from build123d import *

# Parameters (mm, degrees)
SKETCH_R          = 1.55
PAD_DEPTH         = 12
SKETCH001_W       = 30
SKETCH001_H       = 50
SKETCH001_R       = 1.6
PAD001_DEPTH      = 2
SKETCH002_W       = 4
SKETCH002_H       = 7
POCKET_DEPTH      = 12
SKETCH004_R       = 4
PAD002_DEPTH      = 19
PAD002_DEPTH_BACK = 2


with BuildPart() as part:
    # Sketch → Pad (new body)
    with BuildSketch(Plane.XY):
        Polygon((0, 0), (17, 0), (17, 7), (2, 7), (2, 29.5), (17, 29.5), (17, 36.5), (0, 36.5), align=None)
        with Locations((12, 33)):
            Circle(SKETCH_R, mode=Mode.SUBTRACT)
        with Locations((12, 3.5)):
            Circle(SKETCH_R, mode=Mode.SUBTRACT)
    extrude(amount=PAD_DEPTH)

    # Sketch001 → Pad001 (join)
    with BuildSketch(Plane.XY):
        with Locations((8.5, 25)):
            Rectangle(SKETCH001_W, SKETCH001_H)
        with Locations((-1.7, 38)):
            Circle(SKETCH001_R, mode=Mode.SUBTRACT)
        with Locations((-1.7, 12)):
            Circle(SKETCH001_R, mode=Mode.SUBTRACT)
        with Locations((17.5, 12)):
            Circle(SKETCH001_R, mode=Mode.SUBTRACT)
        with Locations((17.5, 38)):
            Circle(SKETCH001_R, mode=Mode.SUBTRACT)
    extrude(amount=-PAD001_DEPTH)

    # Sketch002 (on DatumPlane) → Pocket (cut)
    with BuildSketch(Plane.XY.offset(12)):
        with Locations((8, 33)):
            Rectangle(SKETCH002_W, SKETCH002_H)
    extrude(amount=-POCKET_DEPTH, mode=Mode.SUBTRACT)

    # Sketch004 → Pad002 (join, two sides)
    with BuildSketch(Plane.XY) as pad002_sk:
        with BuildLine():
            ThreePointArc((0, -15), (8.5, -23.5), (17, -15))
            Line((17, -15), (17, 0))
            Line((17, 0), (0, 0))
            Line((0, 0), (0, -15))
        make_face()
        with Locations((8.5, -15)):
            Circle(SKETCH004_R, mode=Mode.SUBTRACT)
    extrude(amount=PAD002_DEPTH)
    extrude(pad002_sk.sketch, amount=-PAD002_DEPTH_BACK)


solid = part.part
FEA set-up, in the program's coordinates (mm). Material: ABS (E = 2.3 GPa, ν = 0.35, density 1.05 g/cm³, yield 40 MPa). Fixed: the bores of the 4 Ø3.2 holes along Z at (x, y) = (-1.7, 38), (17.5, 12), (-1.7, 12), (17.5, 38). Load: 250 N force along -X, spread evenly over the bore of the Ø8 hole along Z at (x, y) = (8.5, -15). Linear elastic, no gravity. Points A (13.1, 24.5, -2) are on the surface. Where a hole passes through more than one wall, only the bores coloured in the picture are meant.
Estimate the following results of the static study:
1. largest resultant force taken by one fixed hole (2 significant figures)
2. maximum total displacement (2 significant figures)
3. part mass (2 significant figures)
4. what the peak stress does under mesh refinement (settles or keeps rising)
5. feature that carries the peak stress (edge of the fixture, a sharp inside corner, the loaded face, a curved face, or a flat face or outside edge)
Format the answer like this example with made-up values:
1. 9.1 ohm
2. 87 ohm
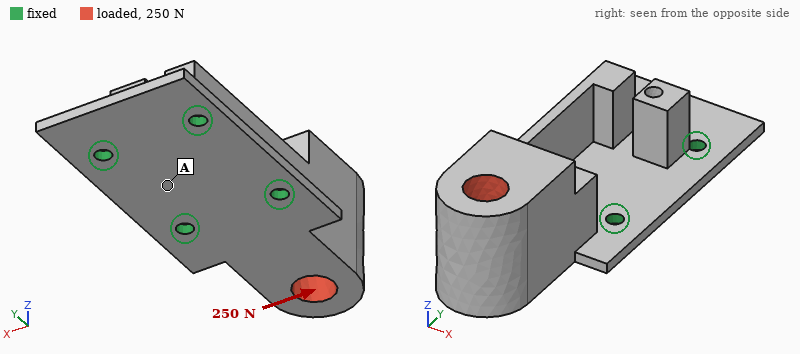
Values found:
1. 370 N
2. 0.79 mm
3. 13 g
4. keeps rising
5. edge of the fixture
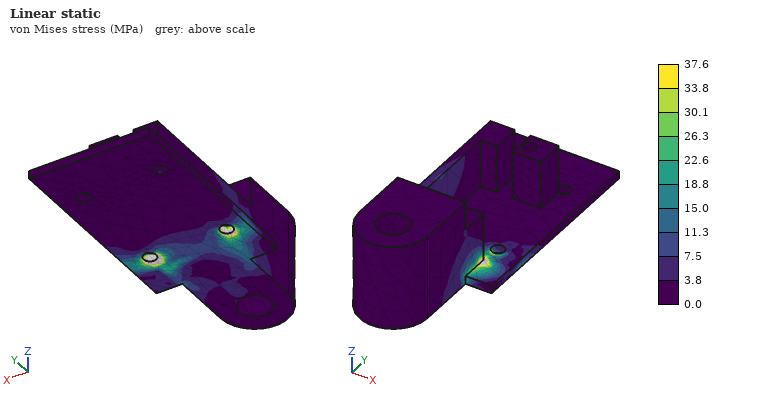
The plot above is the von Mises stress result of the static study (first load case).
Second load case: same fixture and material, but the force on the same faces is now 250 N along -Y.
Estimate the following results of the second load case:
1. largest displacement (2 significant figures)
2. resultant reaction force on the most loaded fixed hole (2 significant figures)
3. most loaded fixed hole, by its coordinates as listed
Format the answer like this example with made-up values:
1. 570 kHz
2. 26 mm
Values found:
1. 0.90 mm
2. 120 N
3. (-1.7, 38)
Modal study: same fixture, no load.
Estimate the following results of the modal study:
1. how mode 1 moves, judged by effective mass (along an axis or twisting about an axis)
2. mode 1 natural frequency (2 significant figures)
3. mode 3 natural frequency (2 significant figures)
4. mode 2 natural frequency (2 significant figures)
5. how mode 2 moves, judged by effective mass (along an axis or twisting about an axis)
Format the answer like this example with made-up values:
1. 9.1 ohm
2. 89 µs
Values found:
1. along Z
2. 740 Hz
3. 2800 Hz
4. 1400 Hz
5. along X
